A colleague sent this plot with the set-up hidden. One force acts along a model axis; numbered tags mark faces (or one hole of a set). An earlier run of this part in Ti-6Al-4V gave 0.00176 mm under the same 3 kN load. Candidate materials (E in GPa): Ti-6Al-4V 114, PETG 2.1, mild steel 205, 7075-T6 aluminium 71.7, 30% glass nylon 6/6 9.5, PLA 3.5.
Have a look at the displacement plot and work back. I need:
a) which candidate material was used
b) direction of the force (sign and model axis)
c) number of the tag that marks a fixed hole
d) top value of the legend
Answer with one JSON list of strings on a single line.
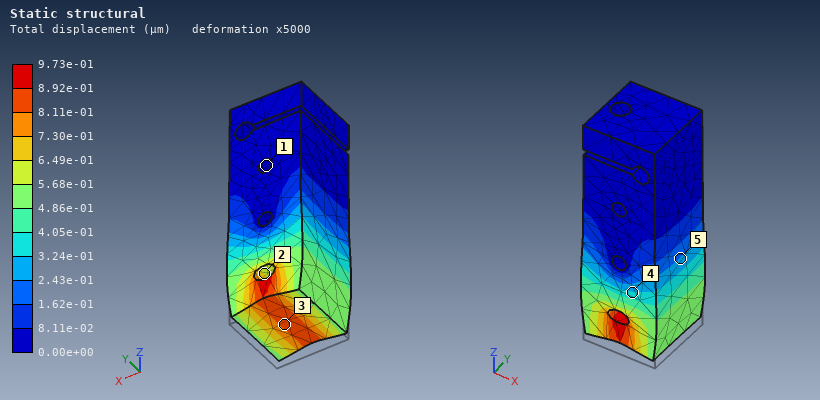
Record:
["mild steel", "+Z", "1", "9.73e-01 µm"]
